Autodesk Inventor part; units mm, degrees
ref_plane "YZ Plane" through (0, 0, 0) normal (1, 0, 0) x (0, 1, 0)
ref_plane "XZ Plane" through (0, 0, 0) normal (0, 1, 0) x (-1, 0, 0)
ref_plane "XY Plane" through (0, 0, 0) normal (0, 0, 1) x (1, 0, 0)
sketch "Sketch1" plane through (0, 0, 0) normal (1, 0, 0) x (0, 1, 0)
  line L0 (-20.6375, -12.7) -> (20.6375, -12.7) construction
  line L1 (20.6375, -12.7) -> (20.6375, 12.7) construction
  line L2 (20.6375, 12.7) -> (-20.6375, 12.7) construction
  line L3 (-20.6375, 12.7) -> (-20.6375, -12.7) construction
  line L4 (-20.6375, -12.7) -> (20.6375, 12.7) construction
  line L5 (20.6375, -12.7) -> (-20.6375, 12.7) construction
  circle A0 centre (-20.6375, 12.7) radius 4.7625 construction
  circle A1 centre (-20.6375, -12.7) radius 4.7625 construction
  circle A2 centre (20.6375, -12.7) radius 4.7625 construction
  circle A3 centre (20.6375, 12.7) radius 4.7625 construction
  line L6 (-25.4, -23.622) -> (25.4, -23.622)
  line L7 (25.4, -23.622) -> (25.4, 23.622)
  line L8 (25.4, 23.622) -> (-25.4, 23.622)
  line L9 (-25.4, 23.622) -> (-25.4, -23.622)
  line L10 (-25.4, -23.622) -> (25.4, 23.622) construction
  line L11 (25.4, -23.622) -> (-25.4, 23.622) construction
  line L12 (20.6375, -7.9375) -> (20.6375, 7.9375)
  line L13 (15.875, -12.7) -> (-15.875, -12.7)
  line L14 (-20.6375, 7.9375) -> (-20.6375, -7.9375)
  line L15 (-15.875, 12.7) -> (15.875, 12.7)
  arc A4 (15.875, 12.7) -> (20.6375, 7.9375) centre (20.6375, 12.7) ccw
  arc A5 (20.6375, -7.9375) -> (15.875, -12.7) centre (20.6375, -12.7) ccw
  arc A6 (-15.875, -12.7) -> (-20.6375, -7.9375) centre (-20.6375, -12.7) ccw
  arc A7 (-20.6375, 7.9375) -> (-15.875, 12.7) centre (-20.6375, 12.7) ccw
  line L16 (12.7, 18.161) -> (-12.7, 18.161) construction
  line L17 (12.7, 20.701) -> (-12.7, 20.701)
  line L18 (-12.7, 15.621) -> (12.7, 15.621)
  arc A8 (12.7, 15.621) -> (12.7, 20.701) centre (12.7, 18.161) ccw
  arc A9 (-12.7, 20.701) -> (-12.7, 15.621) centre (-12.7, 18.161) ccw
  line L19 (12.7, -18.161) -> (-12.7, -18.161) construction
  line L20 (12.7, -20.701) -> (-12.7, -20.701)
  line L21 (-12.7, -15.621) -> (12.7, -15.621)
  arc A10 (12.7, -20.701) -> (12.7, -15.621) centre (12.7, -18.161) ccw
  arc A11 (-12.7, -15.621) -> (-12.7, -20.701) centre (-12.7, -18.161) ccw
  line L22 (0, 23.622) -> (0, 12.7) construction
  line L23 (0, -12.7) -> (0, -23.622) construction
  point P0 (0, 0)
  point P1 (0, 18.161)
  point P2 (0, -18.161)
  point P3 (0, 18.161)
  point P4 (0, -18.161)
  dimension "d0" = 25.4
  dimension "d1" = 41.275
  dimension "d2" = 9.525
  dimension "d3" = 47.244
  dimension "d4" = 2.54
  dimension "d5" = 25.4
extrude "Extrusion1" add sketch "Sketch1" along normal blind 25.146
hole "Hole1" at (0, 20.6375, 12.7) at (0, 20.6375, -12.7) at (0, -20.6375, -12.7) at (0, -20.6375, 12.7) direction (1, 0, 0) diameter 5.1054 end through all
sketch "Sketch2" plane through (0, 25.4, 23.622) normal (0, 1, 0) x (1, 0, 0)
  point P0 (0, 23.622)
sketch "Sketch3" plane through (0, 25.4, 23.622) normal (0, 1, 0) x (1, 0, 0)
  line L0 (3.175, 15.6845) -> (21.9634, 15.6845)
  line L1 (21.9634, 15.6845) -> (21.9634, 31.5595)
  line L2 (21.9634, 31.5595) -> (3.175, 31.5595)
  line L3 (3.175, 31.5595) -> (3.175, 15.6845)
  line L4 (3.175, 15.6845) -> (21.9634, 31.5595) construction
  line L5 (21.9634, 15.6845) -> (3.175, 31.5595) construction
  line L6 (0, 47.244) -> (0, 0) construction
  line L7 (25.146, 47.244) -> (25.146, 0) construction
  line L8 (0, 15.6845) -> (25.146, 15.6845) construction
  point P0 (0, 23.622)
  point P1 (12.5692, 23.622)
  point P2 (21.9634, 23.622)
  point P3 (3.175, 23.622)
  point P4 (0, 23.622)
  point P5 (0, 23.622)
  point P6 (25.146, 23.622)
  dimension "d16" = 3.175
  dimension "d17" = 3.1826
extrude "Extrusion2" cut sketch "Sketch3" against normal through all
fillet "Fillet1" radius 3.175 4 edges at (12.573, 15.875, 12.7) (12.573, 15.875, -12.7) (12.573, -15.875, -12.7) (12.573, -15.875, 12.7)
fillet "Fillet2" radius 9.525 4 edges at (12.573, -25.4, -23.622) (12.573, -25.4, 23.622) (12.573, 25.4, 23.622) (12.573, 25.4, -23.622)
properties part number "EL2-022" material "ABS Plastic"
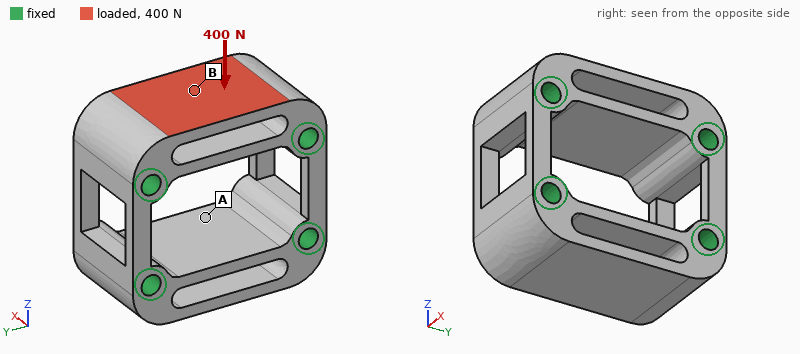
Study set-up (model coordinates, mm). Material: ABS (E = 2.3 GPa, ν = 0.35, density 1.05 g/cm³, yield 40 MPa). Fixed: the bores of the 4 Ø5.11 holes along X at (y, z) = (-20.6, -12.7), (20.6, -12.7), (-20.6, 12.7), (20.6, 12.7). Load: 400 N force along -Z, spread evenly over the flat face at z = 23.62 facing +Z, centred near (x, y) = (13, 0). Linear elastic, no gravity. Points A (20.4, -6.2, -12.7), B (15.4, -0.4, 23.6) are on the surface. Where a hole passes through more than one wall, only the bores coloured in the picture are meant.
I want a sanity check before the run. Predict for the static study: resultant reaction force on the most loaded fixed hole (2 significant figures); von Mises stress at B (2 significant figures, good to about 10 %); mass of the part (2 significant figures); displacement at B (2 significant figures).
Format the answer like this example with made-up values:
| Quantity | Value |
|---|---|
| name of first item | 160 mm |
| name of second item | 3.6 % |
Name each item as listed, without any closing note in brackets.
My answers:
| Quantity | Value |
|---|---|
| resultant reaction force on the most loaded fixed hole | 260 N |
| von Mises stress at B | 14 MPa |
| mass of the part | 23 g |
| displacement at B | 0.27 mm |
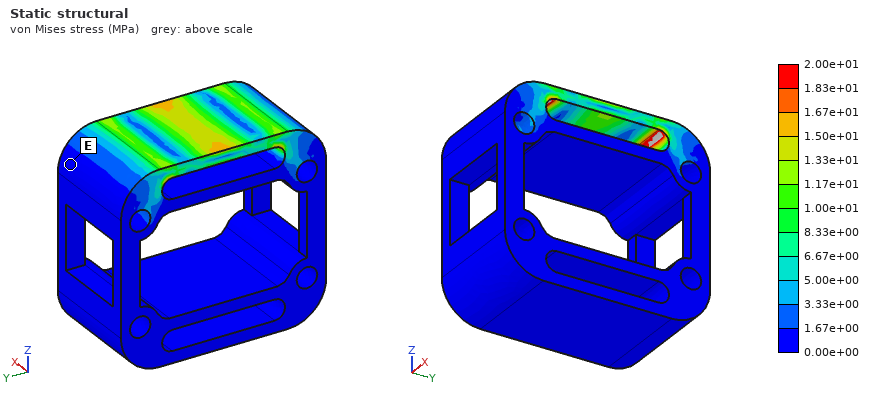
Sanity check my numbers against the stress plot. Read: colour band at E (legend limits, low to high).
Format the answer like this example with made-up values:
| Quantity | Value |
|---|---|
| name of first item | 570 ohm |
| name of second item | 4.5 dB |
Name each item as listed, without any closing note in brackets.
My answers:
| Quantity | Value |
|---|---|
| colour band at E | 0.00e+00 to 1.67e+00 MPa |
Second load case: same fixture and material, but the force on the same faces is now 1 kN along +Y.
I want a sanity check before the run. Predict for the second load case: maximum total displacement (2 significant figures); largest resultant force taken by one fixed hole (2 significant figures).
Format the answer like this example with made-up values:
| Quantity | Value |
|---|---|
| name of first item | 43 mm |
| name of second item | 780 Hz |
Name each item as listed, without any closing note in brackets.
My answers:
| Quantity | Value |
|---|---|
| maximum total displacement | 82 µm |
| largest resultant force taken by one fixed hole | 510 N |
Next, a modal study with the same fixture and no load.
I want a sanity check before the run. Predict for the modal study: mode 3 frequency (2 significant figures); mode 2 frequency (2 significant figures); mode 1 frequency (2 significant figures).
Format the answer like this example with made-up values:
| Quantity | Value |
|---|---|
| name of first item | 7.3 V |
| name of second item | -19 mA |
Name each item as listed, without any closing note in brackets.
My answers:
| Quantity | Value |
|---|---|
| mode 3 frequency | 4700 Hz |
| mode 2 frequency | 4400 Hz |
| mode 1 frequency | 4400 Hz |
